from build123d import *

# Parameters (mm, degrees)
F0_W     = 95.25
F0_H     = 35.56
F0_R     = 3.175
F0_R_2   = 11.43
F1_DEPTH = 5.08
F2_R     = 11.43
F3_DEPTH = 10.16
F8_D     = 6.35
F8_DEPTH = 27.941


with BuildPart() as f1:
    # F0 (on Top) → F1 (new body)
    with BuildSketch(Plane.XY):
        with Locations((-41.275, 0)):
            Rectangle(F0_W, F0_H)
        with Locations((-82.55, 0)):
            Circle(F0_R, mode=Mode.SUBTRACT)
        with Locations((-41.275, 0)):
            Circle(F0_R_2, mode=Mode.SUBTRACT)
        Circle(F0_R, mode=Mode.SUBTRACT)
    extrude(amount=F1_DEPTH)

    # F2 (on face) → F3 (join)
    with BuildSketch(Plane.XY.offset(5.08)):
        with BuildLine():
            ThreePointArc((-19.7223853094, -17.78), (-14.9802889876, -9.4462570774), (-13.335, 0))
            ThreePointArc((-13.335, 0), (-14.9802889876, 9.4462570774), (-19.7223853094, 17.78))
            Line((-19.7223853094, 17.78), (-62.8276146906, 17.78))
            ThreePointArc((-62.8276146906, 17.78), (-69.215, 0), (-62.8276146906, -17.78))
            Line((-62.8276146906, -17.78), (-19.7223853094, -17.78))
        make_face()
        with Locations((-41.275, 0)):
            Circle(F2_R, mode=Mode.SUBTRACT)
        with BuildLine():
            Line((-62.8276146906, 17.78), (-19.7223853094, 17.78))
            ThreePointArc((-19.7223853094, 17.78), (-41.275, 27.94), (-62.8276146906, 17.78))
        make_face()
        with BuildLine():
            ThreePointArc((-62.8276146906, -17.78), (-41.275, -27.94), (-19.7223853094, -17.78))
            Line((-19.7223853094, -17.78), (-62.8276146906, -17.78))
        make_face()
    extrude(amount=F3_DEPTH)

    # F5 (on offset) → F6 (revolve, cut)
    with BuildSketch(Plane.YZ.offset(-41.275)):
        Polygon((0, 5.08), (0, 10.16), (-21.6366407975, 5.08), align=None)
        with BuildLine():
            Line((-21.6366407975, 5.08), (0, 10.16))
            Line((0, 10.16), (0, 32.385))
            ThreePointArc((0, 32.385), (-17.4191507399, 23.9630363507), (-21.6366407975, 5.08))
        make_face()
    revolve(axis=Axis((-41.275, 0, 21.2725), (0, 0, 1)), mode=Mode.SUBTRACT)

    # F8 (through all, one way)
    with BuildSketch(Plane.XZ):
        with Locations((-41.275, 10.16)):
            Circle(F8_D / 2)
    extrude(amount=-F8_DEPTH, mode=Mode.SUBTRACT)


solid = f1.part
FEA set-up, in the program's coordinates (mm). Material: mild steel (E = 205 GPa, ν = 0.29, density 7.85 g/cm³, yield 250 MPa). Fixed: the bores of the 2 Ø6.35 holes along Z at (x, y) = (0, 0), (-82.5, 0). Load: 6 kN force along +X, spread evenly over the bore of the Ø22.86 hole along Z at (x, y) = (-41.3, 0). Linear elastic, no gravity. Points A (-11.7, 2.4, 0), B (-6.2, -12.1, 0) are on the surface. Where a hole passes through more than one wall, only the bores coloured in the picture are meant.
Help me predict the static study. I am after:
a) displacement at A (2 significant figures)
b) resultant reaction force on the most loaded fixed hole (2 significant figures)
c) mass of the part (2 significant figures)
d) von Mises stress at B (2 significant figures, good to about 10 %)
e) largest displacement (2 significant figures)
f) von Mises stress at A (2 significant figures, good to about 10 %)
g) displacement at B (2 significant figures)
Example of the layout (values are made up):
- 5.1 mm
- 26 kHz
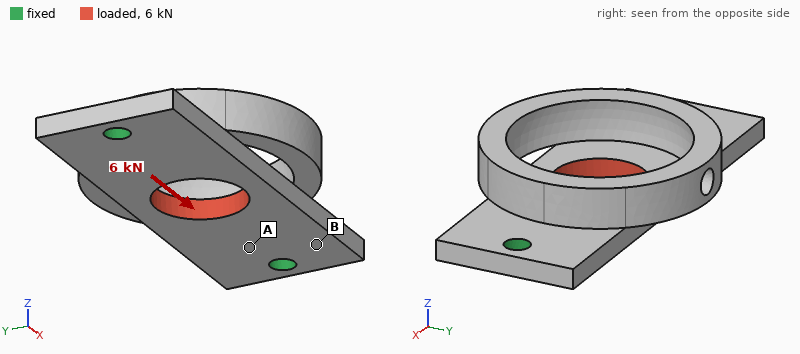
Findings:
- 1.6 µm
- 3.0 kN
- 190 g
- 9.7 MPa
- 4.5 µm
- 28 MPa
- 1.9 µm
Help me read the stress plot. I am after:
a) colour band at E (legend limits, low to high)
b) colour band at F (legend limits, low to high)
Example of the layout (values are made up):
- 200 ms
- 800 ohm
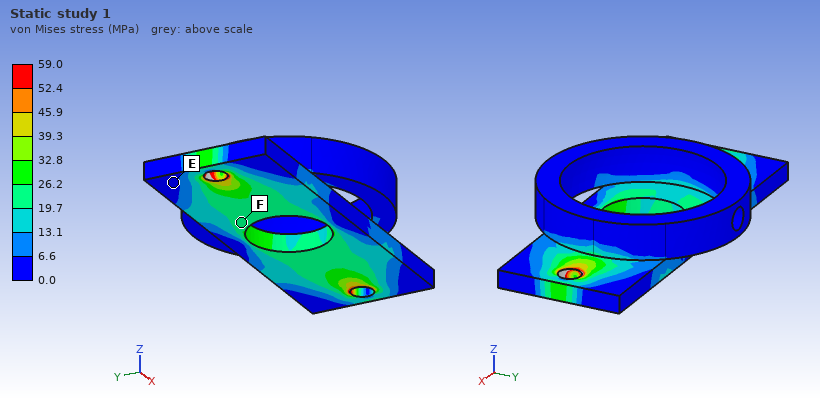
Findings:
- 0.0 to 6.6 MPa
- 19.7 to 26.2 MPa
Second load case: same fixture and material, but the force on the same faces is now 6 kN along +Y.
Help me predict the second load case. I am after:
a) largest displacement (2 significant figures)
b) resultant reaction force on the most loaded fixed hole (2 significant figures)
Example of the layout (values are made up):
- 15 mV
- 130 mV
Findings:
- 19 µm
- 3.0 kN
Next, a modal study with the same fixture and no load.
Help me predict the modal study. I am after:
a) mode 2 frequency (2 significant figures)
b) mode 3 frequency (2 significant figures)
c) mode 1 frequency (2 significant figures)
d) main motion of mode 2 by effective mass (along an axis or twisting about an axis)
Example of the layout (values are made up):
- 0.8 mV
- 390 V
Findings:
- 3900 Hz
- 8900 Hz
- 3200 Hz
- along Z
